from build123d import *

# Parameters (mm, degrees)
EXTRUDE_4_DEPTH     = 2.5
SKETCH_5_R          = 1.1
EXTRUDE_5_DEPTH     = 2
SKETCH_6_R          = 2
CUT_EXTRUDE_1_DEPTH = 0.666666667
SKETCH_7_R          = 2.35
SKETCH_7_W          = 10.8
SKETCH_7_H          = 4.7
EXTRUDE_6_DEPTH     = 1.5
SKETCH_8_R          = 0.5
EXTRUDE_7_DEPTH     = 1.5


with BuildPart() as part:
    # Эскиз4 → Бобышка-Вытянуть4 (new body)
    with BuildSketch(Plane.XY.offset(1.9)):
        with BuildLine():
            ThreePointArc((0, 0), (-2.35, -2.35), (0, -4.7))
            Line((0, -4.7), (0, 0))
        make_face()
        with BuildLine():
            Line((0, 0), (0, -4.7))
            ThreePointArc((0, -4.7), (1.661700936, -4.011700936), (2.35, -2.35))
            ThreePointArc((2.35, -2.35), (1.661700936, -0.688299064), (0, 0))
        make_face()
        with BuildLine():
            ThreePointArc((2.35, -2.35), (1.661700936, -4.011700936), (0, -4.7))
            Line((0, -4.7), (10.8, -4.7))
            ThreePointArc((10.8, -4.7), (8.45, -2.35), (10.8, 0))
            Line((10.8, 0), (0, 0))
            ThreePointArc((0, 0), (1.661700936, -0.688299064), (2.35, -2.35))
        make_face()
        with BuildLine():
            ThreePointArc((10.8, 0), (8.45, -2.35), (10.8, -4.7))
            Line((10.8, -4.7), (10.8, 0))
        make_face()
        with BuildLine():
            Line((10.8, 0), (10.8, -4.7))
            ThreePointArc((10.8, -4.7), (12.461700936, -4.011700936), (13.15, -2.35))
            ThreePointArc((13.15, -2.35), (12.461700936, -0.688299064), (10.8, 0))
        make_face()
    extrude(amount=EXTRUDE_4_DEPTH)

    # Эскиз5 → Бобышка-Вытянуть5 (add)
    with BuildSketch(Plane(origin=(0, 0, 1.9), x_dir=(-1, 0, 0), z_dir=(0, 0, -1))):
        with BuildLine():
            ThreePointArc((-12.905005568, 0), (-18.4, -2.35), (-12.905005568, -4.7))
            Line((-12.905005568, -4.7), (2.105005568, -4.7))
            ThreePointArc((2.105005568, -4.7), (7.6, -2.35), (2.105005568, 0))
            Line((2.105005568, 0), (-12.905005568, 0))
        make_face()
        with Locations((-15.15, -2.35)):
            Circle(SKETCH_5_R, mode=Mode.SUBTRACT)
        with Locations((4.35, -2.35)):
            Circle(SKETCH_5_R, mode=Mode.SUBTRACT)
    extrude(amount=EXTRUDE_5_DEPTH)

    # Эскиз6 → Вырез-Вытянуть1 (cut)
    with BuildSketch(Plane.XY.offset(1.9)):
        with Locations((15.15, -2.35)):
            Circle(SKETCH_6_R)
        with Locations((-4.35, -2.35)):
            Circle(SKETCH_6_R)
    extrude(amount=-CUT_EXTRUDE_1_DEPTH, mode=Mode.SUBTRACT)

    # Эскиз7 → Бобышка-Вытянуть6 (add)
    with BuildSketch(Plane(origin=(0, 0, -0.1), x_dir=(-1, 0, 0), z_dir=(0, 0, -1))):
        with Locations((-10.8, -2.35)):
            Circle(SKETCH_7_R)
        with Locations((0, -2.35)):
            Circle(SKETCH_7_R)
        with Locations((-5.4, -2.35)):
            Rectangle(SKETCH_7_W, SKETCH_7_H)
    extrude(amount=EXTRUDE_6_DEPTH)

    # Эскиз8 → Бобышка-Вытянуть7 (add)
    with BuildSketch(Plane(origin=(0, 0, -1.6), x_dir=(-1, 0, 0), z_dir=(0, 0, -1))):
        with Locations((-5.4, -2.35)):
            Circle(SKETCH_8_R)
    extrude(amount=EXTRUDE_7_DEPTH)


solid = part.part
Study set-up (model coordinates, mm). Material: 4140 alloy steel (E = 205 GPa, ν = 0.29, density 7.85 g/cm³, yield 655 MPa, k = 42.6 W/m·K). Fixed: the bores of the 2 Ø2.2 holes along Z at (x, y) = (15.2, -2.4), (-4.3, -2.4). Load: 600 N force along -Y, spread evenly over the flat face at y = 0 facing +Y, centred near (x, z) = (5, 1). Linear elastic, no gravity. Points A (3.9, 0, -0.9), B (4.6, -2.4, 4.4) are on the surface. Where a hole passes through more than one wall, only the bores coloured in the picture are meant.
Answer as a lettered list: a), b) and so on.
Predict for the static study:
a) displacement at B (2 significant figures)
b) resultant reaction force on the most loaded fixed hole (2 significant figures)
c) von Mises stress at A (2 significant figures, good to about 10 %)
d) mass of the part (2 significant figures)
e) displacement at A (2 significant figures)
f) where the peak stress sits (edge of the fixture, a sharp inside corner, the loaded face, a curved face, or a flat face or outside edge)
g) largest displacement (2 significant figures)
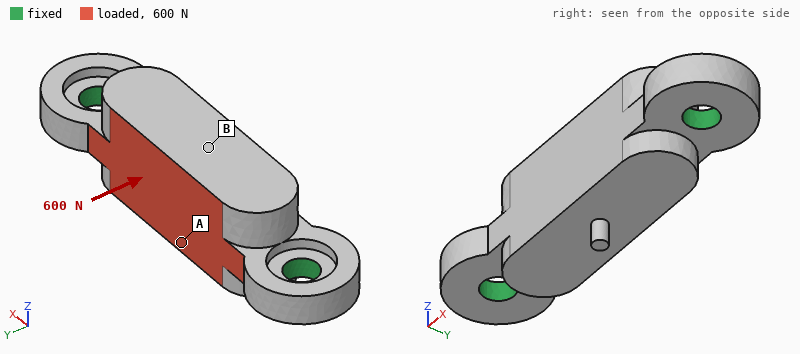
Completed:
a) 7.2 µm
b) 300 N
c) 47 MPa
d) 4.0 g
e) 4.0 µm
f) edge of the fixture
g) 7.5 µm
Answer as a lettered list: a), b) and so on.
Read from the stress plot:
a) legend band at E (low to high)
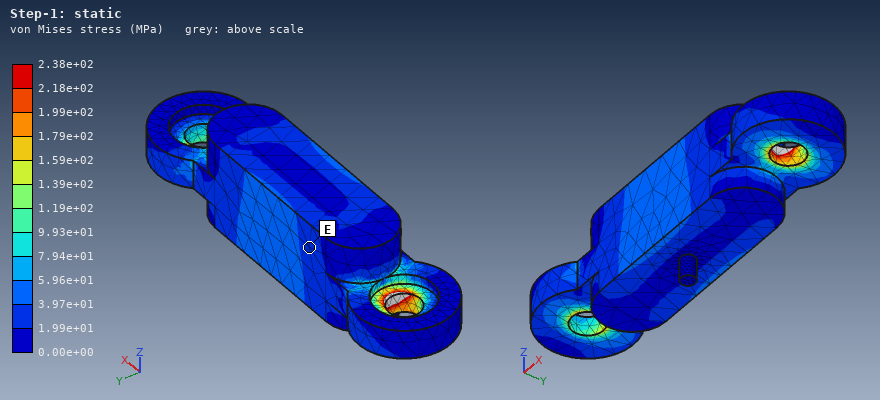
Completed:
a) 1.99e+01 to 3.97e+01 MPa
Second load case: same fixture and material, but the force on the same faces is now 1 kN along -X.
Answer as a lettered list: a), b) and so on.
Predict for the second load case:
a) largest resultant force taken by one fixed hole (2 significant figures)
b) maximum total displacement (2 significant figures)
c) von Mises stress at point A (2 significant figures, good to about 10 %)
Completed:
a) 520 N
b) 1.9 µm
c) 26 MPa
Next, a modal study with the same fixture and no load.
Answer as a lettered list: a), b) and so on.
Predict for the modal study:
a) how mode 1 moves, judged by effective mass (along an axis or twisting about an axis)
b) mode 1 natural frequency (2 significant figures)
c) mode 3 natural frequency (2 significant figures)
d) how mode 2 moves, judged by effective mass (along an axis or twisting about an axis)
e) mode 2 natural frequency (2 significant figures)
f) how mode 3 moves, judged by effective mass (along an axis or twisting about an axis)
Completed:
a) along Y
b) 28 kHz
c) 39 kHz
d) along Z
e) 36 kHz
f) along Y
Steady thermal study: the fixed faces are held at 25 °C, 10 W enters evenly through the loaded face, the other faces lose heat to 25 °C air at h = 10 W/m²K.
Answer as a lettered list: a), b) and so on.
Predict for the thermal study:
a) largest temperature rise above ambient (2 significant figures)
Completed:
a) 55 K
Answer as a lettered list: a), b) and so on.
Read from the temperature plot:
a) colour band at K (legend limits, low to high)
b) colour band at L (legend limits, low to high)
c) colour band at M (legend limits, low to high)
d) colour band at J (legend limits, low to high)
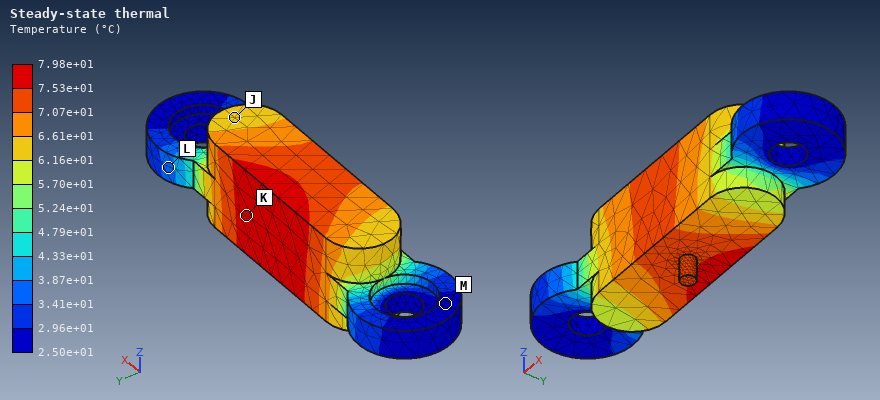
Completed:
a) 7.53e+01 to 7.98e+01 °C
b) 3.41e+01 to 3.87e+01 °C
c) 2.50e+01 to 2.96e+01 °C
d) 6.16e+01 to 6.61e+01 °C
